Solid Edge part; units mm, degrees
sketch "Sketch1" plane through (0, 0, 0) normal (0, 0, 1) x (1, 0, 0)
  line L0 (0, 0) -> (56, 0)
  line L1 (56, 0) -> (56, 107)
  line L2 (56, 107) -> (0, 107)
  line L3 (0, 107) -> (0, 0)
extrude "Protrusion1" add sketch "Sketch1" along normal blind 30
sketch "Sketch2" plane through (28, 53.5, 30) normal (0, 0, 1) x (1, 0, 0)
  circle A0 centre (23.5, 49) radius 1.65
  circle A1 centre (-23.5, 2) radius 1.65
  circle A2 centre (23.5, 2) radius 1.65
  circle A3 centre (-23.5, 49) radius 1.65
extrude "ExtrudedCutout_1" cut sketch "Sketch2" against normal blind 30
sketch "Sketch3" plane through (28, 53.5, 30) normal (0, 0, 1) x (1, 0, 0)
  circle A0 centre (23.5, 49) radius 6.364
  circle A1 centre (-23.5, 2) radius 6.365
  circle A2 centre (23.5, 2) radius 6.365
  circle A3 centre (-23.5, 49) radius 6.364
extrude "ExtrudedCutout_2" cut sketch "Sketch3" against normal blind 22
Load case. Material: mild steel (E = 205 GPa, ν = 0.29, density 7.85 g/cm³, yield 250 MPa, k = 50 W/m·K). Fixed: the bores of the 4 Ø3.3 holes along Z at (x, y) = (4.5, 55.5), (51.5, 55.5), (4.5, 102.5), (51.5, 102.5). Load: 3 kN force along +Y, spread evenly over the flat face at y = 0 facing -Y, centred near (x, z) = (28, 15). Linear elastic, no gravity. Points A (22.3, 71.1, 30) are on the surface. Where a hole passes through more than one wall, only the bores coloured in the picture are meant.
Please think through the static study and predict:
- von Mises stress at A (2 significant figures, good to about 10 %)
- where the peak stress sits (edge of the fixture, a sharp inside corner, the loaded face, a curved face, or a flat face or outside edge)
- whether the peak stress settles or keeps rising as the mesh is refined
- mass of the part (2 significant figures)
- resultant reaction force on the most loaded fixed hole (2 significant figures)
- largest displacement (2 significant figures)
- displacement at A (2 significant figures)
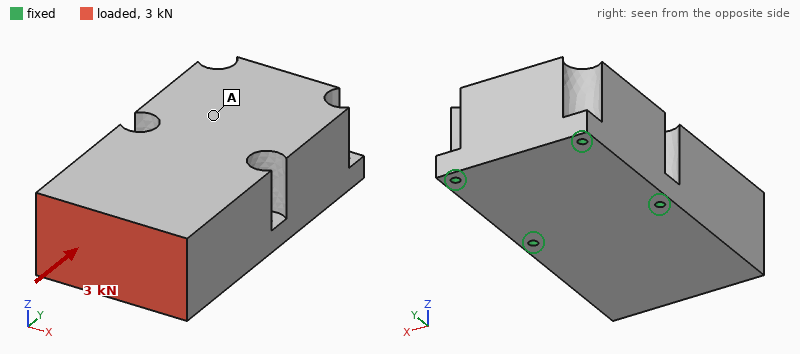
2.2 MPa
edge of the fixture
keeps rising
1.3 kg
1.0 kN
3.1 µm
0.99 µm
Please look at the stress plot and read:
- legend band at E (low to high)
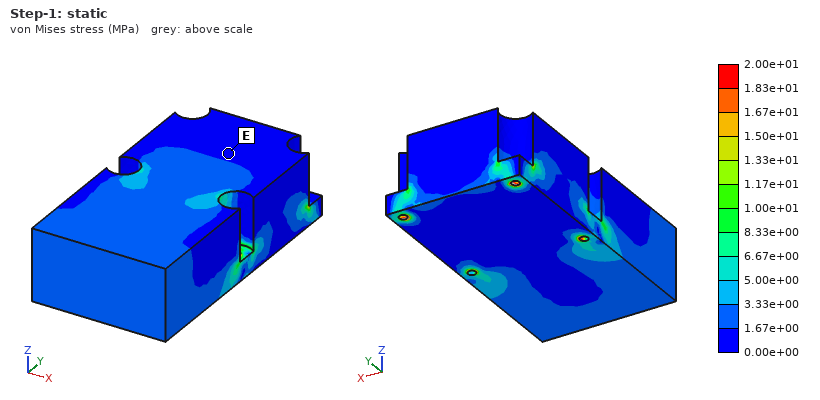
0.00e+00 to 1.67e+00 MPa
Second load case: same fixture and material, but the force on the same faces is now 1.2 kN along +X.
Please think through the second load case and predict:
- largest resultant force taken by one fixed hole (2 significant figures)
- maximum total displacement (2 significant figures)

1.3 kN
3.3 µm
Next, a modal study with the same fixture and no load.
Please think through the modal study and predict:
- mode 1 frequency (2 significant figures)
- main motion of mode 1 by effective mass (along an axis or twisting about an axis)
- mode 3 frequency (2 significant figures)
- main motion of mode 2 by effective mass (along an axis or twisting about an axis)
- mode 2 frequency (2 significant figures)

3300 Hz
along Z
8000 Hz
along X
5900 Hz
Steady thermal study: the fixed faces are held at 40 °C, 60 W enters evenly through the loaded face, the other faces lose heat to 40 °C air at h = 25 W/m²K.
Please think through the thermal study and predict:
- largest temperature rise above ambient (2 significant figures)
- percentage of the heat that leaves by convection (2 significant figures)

55 K
20 %
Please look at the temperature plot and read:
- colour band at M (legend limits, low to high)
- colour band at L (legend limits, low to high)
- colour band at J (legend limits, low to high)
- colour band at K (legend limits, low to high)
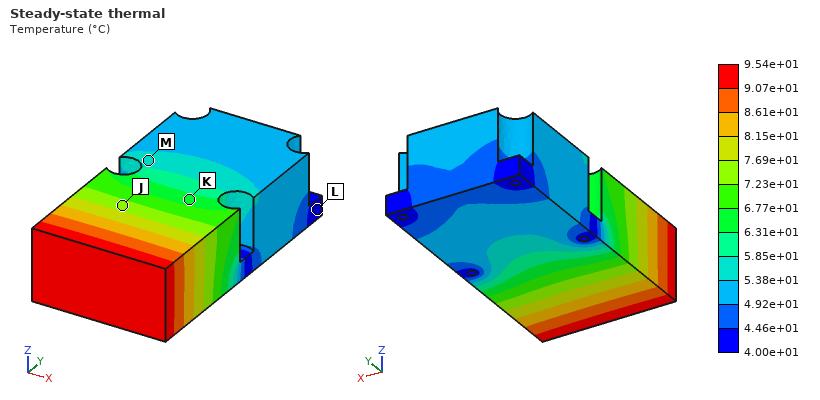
5.38e+01 to 5.85e+01 °C
4.00e+01 to 4.46e+01 °C
7.23e+01 to 7.69e+01 °C
6.31e+01 to 6.77e+01 °C
